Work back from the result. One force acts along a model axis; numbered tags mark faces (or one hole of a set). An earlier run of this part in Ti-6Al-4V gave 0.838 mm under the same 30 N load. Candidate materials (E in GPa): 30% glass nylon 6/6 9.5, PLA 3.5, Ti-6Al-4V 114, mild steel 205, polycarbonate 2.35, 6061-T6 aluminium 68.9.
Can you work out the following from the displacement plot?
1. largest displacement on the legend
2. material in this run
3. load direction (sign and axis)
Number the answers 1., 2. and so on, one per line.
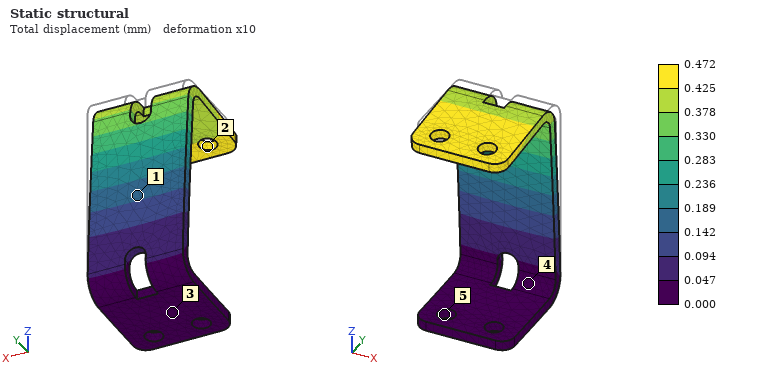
1. 0.472 mm
2. mild steel
3. -Y
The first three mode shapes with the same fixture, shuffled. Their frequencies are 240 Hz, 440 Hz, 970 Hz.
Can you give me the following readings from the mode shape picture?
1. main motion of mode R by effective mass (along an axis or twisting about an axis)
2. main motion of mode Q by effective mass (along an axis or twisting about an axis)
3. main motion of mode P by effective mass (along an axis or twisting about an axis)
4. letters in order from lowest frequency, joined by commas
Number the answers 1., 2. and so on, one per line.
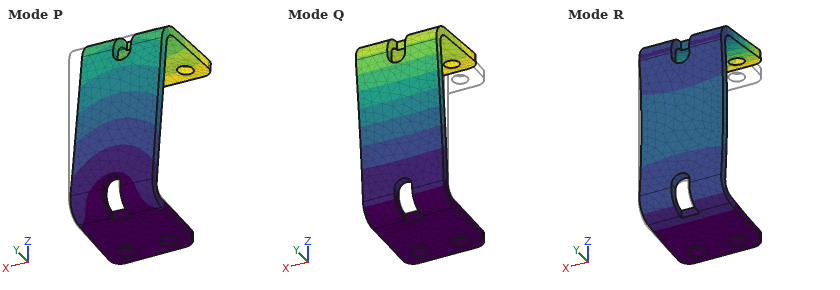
1. along Z
2. along Y
3. along X
4. Q, P, R
